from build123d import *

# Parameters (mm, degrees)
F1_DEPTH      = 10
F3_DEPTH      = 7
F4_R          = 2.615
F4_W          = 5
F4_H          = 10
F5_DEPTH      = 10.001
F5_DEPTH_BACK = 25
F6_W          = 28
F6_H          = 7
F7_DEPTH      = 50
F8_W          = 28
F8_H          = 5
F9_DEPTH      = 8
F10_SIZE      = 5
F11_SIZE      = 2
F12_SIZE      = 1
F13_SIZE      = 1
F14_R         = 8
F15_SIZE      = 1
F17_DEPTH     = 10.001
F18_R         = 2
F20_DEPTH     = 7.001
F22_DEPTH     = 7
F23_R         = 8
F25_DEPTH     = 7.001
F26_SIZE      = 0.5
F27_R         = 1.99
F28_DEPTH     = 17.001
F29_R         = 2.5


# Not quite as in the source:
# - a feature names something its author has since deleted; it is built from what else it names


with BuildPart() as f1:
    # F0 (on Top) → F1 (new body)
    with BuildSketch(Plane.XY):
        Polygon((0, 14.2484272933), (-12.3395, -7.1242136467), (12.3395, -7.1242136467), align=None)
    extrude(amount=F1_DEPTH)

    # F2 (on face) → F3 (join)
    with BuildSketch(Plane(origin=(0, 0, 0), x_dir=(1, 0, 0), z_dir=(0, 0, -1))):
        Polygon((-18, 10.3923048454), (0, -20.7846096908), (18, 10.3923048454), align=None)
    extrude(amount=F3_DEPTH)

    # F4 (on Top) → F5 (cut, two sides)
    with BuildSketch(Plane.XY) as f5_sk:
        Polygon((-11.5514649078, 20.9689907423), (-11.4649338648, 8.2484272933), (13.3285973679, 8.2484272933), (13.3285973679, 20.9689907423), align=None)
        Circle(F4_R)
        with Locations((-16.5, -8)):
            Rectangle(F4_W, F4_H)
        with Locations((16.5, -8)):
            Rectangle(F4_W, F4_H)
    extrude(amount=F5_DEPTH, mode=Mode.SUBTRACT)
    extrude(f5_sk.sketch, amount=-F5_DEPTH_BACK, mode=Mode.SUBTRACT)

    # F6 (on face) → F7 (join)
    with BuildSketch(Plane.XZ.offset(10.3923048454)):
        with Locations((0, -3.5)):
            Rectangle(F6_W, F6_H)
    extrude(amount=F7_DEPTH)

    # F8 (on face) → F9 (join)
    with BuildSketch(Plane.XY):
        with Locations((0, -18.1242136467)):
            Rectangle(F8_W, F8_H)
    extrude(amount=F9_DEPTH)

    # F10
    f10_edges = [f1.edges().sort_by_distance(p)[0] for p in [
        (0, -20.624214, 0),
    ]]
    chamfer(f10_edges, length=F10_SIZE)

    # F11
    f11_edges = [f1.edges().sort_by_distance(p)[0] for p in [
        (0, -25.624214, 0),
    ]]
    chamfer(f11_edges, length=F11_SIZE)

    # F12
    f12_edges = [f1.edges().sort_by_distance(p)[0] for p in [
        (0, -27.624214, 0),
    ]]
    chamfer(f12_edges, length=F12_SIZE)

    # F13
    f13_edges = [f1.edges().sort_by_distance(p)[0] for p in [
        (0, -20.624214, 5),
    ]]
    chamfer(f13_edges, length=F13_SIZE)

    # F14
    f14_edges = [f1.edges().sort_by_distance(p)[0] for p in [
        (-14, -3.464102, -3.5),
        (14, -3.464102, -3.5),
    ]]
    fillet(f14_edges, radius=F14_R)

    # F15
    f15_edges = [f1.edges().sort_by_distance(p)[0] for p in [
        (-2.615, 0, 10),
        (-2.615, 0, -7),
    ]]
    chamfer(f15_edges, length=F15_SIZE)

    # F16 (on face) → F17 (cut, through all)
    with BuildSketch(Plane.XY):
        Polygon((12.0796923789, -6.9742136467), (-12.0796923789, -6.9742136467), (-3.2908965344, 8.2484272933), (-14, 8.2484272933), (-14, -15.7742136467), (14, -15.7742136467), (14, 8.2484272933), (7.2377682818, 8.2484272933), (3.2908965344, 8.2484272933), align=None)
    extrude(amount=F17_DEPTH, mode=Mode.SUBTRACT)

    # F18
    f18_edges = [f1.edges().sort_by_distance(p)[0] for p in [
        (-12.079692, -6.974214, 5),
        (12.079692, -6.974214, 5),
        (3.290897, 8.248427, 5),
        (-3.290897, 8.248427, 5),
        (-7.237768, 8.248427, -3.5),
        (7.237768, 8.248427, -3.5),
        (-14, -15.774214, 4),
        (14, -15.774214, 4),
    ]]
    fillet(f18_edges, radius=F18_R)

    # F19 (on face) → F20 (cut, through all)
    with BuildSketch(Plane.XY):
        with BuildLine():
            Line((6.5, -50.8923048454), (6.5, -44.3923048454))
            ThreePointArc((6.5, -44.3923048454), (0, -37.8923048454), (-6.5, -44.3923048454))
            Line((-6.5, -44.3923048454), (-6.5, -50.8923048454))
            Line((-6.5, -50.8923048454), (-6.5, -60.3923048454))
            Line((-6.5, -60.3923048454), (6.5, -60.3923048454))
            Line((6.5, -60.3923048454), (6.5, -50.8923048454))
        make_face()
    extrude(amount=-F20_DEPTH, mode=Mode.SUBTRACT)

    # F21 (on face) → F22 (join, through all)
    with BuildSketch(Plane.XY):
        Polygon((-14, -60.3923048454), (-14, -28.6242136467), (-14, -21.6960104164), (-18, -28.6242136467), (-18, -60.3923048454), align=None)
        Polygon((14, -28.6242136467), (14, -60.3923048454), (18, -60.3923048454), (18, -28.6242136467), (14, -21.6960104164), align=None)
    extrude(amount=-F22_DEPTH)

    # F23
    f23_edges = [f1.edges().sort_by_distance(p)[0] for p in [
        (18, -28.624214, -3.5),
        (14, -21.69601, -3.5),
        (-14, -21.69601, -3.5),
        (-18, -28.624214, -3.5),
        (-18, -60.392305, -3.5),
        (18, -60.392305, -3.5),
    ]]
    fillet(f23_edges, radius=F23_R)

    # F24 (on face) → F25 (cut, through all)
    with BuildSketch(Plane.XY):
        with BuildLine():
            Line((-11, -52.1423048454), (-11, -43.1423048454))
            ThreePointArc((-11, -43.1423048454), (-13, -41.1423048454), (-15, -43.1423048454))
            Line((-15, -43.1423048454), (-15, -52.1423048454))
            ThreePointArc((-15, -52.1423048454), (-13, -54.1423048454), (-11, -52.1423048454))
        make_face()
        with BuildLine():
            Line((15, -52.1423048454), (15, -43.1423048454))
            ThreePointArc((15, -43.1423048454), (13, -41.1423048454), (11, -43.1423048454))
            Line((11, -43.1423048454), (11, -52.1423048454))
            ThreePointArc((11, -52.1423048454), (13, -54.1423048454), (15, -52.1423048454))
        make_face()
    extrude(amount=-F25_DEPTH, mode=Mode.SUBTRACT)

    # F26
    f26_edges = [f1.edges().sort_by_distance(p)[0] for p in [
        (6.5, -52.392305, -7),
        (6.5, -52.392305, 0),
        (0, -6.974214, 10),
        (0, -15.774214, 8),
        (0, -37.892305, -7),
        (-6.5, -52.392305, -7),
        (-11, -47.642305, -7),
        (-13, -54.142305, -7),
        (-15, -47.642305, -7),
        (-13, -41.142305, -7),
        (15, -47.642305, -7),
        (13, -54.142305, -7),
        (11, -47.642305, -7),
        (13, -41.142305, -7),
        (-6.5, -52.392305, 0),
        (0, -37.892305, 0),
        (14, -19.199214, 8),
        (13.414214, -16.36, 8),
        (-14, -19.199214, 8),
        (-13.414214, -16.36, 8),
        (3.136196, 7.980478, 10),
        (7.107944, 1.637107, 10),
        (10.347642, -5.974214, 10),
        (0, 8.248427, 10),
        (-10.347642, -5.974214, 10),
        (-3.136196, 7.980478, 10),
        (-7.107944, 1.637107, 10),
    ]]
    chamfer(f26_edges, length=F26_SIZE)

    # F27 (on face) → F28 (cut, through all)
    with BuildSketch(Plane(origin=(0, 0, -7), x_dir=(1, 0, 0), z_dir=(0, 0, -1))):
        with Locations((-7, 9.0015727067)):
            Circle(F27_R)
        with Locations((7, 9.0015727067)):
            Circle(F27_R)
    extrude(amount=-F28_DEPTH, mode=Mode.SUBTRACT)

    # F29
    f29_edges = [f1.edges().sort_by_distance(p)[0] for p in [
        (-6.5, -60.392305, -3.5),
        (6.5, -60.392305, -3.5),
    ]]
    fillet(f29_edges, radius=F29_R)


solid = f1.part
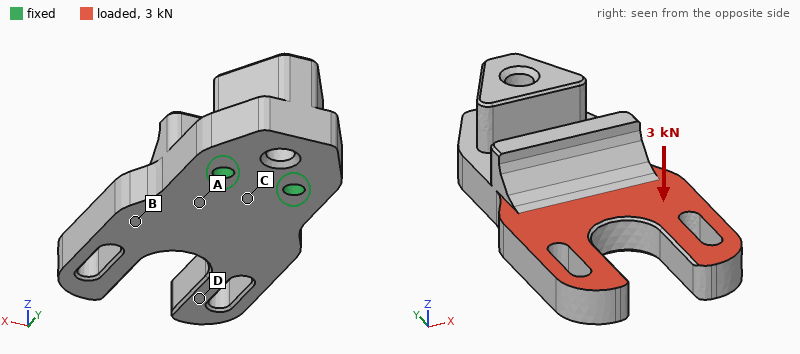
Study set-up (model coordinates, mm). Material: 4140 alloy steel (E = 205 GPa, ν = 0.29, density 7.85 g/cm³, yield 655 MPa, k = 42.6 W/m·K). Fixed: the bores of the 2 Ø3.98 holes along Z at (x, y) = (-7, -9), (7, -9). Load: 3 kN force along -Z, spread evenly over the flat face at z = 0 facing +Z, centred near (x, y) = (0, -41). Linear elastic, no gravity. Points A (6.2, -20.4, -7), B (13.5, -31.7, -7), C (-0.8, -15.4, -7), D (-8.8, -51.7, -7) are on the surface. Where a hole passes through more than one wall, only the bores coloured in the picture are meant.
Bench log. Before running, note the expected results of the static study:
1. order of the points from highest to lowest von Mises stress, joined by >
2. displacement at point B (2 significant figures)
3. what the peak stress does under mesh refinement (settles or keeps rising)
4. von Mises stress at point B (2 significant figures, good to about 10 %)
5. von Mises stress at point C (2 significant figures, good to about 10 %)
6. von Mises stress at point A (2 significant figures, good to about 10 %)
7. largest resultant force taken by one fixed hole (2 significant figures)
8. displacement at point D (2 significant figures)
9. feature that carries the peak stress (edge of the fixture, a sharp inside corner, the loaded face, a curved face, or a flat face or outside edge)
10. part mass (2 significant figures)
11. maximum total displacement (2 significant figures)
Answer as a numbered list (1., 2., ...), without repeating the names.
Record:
1. C > A > B > D
2. 0.10 mm
3. keeps rising
4. 97 MPa
5. 260 MPa
6. 160 MPa
7. 1.5 kN
8. 0.25 mm
9. edge of the fixture
10. 120 g
11. 0.33 mm
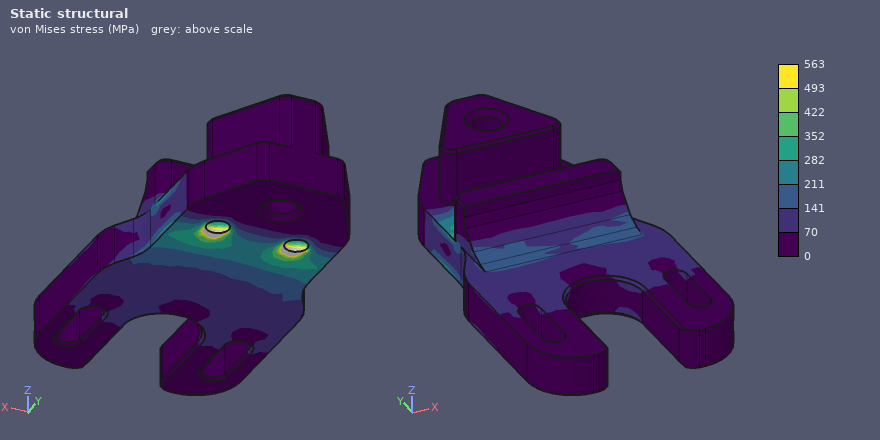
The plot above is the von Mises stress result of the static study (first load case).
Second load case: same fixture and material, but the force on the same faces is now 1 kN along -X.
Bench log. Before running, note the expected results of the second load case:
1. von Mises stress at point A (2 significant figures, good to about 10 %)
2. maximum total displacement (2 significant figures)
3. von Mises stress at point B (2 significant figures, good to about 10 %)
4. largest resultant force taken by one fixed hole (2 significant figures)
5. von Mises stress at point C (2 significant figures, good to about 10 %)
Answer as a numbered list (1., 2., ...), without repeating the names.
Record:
1. 11 MPa
2. 18 µm
3. 10 MPa
4. 2.0 kN
5. 12 MPa
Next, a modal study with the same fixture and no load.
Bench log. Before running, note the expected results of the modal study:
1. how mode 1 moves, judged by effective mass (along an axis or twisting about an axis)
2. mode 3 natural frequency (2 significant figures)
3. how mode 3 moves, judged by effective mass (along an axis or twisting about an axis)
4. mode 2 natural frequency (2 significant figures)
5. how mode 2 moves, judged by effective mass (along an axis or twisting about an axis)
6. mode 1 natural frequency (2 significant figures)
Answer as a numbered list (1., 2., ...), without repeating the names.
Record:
1. along Z
2. 7200 Hz
3. along X
4. 5400 Hz
5. twisting about Y
6. 2900 Hz
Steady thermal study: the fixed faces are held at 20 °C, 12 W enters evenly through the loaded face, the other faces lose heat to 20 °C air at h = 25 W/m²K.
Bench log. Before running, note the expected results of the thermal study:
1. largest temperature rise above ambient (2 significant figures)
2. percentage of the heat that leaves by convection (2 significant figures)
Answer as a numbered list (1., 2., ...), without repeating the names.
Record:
1. 38 K
2. 18 %
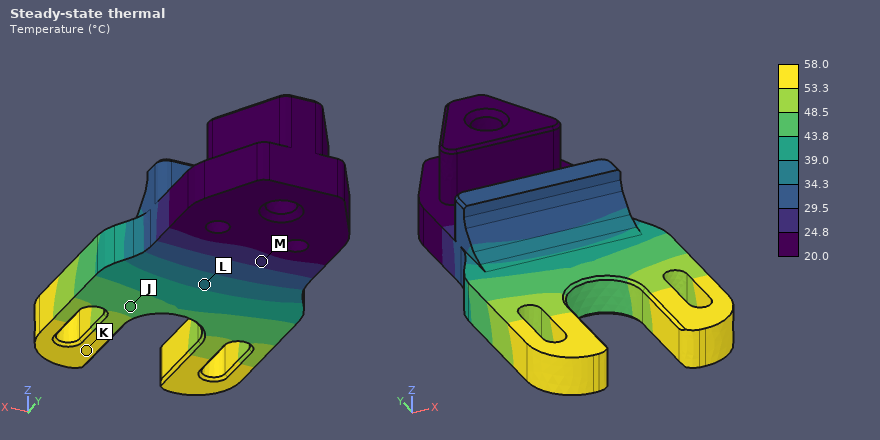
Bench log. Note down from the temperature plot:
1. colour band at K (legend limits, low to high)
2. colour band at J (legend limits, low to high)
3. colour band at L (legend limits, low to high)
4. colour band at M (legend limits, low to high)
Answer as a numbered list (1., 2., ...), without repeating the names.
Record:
1. 53.3 to 58.0 °C
2. 43.8 to 48.5 °C
3. 34.3 to 39.0 °C
4. 24.8 to 29.5 °C
